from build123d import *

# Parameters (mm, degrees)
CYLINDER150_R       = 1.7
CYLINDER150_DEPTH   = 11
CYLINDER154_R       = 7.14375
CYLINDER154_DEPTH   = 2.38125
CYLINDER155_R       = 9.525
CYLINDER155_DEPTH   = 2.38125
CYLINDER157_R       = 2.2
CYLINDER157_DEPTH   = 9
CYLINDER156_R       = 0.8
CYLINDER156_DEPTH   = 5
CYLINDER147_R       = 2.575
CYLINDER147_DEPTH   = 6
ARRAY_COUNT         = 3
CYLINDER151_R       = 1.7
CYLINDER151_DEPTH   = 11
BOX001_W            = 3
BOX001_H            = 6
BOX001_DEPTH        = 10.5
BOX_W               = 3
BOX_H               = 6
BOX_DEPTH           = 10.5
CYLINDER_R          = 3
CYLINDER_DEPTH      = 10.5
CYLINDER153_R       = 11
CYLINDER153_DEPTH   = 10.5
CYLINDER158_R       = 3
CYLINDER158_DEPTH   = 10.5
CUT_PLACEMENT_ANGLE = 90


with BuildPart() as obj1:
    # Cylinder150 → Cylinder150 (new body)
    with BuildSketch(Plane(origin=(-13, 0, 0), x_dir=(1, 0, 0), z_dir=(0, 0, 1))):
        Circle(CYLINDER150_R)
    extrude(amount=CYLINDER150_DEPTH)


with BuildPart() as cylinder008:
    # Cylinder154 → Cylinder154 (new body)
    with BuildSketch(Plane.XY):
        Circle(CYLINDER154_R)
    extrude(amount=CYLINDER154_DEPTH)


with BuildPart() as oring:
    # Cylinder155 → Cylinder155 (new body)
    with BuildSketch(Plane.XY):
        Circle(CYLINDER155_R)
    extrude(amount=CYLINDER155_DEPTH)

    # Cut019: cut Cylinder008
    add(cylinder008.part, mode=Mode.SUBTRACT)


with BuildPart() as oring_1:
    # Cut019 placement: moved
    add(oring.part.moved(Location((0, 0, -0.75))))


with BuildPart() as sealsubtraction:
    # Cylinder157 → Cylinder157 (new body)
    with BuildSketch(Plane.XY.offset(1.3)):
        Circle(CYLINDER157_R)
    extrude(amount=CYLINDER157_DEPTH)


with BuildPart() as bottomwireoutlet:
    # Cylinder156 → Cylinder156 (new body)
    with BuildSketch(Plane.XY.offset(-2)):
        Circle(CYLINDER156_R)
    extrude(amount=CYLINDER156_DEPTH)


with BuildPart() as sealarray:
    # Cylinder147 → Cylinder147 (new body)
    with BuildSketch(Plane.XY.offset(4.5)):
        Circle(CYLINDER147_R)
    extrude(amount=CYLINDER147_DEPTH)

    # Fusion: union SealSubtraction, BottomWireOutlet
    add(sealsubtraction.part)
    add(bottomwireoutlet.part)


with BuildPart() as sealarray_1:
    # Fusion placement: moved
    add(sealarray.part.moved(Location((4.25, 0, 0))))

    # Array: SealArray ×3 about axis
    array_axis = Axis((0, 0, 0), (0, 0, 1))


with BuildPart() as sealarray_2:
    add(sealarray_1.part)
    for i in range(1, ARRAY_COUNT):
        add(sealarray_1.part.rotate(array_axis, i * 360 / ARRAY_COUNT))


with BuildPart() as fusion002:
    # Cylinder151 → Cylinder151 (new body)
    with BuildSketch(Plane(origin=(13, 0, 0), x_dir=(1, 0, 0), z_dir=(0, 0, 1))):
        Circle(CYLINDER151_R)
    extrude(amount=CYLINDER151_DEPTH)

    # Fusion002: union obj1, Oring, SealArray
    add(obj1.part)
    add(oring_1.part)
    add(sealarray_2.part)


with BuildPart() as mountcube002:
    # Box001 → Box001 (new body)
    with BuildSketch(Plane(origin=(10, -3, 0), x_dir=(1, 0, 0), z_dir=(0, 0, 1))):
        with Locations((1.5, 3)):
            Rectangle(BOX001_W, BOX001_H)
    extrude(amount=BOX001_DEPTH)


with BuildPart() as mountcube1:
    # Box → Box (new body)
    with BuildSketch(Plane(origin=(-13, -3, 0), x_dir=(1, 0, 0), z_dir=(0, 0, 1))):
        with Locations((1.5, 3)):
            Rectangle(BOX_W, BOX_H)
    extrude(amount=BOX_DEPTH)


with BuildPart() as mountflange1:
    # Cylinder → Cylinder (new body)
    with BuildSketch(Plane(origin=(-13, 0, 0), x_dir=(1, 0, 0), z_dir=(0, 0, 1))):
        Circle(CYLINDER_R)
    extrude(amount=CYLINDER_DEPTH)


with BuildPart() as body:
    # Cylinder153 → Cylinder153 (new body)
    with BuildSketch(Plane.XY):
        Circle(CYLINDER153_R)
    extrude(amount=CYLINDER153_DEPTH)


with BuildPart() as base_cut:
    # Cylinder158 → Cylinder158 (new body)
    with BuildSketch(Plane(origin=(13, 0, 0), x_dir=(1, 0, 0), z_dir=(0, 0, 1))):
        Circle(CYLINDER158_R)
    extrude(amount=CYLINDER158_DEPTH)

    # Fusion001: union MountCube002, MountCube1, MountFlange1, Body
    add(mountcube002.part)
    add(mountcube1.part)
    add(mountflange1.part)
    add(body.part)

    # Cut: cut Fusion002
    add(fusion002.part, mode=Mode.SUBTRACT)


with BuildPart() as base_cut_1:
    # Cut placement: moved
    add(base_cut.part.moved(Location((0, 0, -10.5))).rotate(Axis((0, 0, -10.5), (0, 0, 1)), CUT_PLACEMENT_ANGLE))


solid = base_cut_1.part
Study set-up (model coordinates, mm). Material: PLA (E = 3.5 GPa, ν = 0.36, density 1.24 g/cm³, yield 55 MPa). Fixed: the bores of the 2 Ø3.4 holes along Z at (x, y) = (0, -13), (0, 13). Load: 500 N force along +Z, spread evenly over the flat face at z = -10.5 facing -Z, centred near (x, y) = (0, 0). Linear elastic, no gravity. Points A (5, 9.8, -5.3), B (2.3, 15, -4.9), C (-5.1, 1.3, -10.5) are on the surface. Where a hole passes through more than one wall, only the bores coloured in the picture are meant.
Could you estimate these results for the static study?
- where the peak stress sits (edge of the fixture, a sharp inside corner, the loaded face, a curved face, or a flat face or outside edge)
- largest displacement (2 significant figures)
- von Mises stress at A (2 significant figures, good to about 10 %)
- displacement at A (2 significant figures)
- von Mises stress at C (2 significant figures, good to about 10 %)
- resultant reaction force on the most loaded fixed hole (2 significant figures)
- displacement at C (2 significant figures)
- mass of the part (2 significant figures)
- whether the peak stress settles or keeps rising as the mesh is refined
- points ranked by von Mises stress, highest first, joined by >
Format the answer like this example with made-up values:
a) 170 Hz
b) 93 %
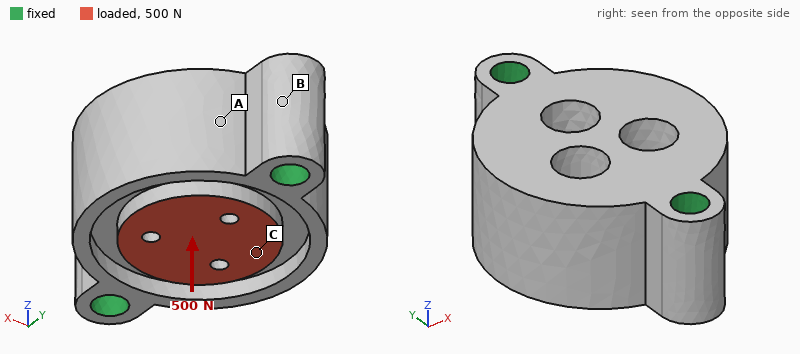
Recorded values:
a) edge of the fixture
b) 41 µm
c) 4.8 MPa
d) 14 µm
e) 3.5 MPa
f) 260 N
g) 34 µm
h) 4.5 g
i) keeps rising
j) A > C > B
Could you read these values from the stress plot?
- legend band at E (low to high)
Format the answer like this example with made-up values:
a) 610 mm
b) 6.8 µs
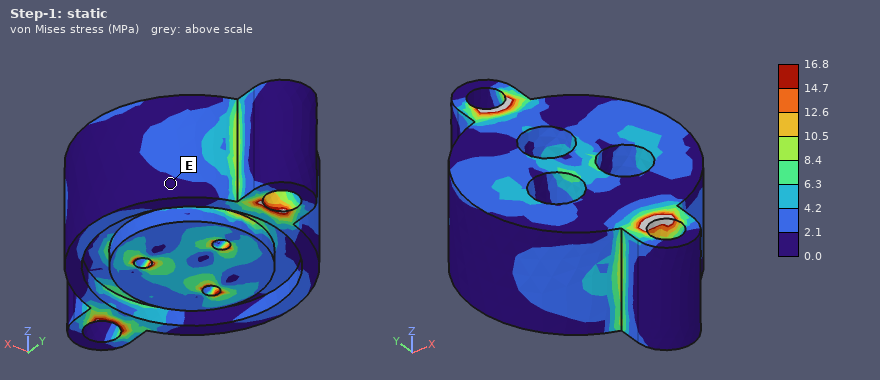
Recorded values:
a) 0.0 to 2.1 MPa
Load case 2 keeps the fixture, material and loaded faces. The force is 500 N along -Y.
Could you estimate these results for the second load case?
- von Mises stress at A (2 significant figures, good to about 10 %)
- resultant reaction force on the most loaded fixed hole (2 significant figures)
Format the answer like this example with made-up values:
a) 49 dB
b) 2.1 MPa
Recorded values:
a) 3.2 MPa
b) 290 N
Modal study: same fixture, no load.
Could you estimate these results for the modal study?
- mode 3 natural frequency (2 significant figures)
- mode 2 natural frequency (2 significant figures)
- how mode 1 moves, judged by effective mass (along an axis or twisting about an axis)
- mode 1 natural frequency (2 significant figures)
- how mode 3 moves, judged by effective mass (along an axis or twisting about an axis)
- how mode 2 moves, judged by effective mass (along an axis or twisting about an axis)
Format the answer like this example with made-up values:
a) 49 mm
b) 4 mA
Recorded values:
a) 14 kHz
b) 11 kHz
c) twisting about Y
d) 8700 Hz
e) along X
f) along Z
